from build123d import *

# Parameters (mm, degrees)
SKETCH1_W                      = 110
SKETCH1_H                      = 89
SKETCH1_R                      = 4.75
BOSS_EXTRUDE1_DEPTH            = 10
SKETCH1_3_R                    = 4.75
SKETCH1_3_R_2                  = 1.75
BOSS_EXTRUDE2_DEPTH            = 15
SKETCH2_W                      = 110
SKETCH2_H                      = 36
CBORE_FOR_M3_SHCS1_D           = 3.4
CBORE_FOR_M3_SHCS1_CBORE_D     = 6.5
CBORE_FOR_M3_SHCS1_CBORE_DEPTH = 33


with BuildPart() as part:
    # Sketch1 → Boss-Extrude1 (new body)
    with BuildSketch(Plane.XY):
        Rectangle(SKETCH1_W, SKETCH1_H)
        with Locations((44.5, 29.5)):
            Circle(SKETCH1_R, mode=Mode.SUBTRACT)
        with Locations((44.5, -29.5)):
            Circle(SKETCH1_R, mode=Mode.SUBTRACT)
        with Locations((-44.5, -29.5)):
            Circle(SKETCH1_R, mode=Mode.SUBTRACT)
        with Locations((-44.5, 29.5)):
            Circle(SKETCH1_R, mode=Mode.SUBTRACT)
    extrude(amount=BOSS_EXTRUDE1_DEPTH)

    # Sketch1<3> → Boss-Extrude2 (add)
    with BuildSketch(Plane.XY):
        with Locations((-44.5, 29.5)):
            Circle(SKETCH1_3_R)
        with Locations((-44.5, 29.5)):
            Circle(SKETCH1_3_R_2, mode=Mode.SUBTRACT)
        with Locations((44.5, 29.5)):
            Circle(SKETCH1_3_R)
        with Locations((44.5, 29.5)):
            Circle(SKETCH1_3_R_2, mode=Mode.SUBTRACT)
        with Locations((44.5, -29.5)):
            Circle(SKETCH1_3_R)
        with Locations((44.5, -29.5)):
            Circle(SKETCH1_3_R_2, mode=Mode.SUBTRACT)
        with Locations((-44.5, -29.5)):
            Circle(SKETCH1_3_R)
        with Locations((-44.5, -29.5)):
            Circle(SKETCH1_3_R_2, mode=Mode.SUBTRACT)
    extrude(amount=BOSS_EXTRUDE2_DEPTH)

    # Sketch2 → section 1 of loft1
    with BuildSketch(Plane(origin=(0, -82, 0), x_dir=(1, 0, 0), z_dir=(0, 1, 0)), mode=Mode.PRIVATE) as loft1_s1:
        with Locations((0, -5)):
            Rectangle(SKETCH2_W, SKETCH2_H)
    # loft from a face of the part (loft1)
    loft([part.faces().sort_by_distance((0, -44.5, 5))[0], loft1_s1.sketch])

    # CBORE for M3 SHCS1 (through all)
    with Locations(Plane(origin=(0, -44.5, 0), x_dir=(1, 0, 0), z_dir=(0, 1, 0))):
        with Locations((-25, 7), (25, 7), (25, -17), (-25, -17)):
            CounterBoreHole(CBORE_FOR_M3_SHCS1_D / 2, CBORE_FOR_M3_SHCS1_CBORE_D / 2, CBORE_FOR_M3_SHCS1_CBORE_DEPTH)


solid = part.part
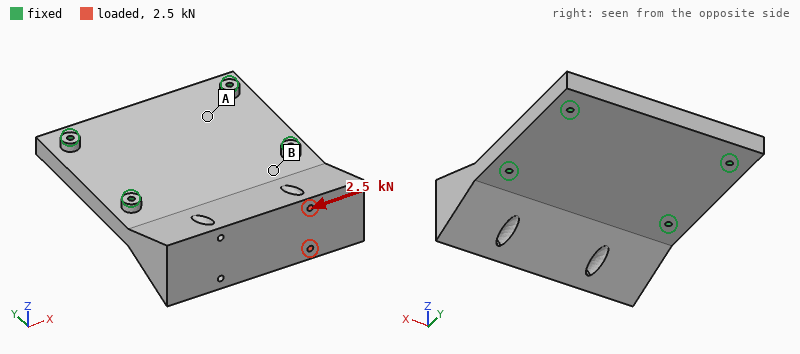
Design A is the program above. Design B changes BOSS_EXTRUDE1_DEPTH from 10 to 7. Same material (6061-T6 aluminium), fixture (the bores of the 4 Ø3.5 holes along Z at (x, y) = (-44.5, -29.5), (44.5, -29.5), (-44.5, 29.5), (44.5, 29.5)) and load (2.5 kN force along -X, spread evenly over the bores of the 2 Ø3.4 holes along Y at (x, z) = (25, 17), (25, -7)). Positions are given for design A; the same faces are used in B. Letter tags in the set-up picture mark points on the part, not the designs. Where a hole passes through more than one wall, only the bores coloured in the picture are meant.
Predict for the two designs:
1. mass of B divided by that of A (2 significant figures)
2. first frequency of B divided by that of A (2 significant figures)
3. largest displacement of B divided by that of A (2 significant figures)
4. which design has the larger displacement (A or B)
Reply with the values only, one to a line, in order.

0.82
0.65
1.3
B
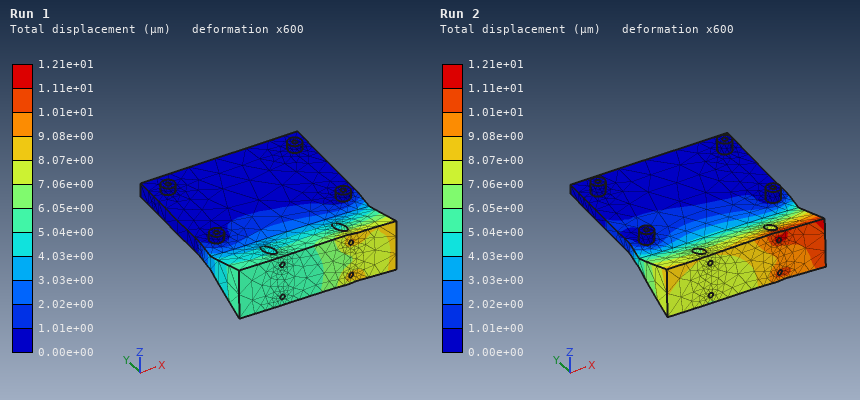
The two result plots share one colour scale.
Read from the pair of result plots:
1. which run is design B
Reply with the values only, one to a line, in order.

Run 2
